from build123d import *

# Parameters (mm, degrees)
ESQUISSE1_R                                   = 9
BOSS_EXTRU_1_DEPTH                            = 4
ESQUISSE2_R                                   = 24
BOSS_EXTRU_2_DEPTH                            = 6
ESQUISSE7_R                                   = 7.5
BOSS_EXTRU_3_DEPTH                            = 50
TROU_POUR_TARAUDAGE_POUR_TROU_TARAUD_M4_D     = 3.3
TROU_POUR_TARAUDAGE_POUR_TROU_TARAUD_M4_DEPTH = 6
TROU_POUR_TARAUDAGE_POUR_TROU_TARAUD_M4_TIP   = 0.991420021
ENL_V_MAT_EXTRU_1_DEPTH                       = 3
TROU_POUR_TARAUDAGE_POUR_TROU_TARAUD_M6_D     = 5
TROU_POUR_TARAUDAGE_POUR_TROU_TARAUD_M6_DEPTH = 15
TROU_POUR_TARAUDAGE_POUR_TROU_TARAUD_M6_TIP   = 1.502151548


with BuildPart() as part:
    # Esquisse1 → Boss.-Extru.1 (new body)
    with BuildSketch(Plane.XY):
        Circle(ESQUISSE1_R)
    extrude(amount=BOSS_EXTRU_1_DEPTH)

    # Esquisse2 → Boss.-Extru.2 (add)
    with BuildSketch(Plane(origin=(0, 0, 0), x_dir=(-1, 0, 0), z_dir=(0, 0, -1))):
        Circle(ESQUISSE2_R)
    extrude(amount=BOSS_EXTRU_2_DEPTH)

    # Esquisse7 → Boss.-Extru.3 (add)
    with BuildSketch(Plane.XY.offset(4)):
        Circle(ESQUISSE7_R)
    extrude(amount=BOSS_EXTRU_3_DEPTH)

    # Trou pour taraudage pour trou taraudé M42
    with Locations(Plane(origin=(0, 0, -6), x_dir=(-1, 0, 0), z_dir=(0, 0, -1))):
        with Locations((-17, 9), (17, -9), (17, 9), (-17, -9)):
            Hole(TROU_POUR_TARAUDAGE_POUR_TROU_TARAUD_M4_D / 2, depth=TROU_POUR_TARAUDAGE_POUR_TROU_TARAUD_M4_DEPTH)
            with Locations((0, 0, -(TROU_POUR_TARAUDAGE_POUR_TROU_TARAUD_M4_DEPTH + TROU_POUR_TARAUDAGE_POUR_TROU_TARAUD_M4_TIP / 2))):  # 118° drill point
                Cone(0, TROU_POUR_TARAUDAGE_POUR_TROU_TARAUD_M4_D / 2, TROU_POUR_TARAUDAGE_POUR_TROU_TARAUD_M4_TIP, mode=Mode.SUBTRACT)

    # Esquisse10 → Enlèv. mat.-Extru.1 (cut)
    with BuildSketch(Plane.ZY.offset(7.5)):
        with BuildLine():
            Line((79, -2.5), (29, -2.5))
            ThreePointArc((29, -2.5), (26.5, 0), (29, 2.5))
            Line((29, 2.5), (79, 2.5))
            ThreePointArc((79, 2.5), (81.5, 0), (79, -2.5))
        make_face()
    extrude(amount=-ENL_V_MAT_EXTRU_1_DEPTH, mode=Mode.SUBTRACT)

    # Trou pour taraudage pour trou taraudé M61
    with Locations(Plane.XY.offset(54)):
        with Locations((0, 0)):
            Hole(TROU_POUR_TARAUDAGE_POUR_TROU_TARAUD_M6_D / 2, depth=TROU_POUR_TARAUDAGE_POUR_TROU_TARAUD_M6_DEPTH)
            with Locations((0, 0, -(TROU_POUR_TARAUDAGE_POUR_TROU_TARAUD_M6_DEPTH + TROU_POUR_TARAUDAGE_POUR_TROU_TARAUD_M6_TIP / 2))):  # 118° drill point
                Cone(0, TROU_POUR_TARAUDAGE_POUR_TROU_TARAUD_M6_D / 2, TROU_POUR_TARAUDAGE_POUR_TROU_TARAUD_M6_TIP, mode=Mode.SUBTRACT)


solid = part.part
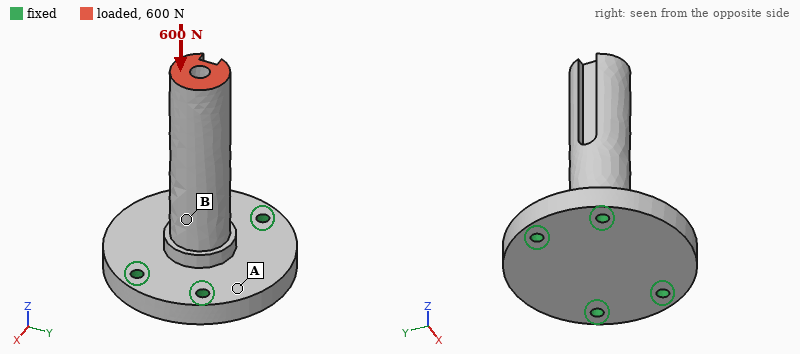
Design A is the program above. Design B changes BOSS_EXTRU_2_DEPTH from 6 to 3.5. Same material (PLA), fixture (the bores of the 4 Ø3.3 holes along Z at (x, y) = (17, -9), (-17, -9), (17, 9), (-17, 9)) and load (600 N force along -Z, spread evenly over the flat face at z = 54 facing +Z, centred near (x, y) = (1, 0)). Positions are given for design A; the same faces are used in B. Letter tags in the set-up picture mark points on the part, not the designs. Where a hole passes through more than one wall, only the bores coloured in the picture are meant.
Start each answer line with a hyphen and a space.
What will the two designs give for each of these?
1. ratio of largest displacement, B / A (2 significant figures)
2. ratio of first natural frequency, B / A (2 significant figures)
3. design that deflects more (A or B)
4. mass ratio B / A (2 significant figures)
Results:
- 1.8
- 0.72
- B
- 0.78
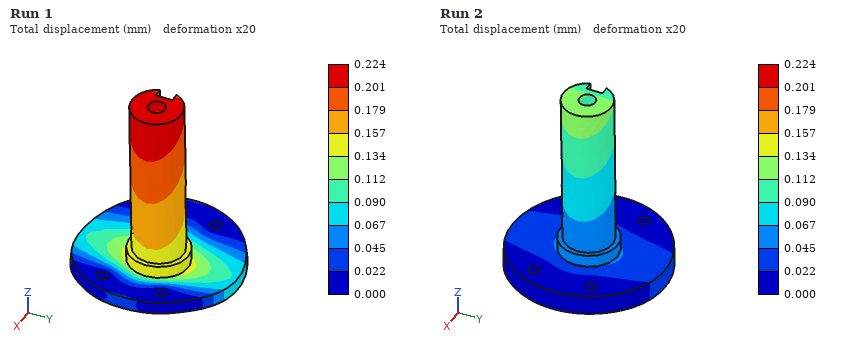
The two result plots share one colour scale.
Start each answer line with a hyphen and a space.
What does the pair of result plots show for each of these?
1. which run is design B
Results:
- Run 1
